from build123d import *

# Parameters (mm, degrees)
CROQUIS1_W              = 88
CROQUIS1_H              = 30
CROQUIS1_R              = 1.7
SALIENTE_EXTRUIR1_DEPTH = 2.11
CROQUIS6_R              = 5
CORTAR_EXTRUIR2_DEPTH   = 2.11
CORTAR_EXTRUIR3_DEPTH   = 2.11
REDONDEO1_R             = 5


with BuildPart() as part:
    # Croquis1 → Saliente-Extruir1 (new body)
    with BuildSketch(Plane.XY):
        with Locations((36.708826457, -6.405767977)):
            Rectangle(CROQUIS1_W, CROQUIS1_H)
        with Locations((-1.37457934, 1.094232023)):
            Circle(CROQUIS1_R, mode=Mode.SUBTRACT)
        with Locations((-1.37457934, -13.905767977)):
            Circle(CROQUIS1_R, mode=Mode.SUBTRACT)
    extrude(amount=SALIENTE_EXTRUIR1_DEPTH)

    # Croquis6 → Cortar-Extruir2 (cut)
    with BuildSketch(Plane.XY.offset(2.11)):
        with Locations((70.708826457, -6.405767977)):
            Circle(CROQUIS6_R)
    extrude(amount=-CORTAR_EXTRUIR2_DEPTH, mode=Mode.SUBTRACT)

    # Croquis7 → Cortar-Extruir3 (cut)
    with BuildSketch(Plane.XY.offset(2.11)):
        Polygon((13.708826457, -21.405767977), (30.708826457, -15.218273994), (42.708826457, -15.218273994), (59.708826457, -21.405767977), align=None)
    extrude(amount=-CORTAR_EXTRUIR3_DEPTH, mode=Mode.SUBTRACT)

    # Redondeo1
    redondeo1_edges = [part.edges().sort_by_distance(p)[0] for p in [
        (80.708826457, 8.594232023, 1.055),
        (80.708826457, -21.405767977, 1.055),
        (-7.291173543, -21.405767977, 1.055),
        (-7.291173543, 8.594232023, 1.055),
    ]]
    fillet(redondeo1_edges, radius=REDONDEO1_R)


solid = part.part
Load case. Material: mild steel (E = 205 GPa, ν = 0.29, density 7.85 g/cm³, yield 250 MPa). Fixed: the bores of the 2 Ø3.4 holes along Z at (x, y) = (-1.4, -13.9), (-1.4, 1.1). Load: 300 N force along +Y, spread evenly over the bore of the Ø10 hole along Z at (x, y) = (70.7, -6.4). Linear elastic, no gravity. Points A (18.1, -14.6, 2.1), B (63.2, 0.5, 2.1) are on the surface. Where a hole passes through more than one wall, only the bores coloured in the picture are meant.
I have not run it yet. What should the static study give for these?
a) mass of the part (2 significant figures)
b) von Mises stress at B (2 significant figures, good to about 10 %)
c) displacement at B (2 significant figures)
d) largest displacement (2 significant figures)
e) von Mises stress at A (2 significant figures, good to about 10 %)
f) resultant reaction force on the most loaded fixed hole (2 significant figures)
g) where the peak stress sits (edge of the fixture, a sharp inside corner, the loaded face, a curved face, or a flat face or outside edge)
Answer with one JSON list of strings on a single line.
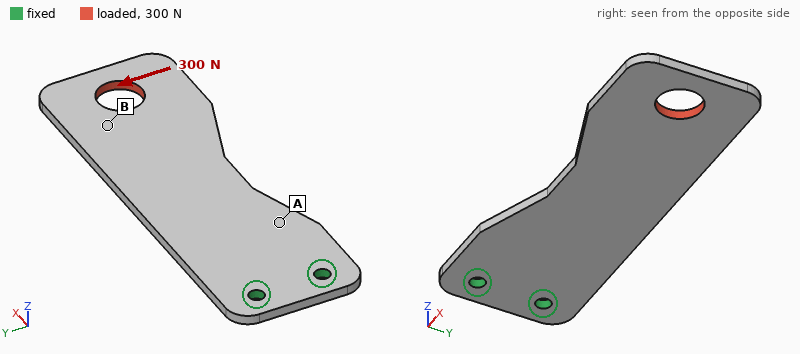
["39 g", "9.2 MPa", "55 µm", "79 µm", "40 MPa", "1.3 kN", "edge of the fixture"]
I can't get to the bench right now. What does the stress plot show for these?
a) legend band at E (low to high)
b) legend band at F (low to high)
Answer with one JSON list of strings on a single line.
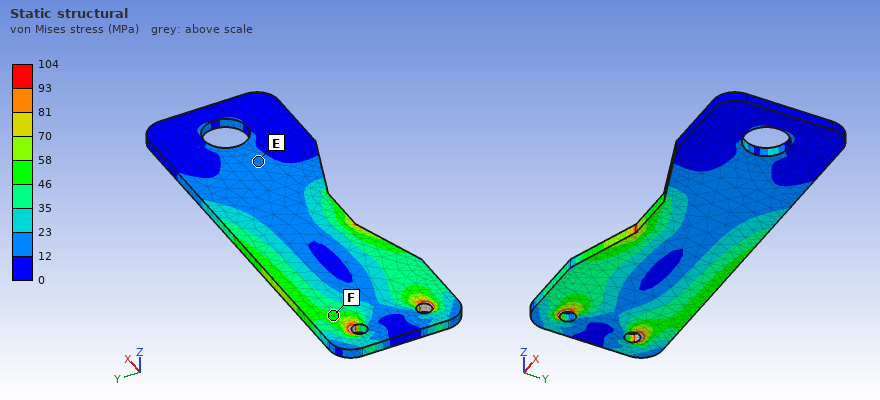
["12 to 23 MPa", "46 to 58 MPa"]
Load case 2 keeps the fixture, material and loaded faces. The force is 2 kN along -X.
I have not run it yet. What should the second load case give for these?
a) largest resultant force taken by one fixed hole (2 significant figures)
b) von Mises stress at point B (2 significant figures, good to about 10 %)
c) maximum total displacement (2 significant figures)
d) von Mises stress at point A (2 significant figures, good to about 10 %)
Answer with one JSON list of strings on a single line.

["1.0 kN", "46 MPa", "24 µm", "39 MPa"]
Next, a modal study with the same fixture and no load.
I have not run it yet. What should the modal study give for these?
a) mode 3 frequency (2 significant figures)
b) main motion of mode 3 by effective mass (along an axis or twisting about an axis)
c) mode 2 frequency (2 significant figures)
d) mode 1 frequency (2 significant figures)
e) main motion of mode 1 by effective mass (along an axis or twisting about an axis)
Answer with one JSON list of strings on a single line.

["1700 Hz", "along Z", "1500 Hz", "270 Hz", "along Z"]
